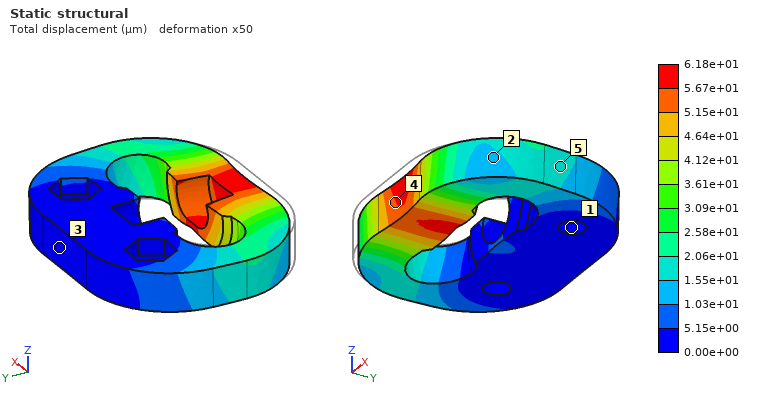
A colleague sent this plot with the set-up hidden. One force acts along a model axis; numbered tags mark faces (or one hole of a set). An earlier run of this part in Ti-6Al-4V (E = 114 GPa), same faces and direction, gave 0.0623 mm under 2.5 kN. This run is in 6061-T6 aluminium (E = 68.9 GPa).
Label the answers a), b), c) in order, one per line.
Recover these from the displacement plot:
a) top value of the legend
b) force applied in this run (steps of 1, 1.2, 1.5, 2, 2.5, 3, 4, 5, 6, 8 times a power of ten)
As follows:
a) 6.18e+01 µm
b) 1.5 kN
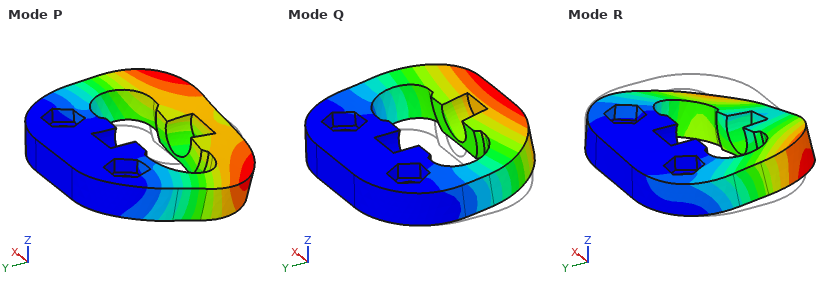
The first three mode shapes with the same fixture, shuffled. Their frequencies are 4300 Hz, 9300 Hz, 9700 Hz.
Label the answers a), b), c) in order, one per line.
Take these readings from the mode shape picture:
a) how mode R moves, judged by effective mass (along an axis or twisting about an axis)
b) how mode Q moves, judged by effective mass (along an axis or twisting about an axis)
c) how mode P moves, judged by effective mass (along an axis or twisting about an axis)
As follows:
a) along X
b) along Z
c) along X
